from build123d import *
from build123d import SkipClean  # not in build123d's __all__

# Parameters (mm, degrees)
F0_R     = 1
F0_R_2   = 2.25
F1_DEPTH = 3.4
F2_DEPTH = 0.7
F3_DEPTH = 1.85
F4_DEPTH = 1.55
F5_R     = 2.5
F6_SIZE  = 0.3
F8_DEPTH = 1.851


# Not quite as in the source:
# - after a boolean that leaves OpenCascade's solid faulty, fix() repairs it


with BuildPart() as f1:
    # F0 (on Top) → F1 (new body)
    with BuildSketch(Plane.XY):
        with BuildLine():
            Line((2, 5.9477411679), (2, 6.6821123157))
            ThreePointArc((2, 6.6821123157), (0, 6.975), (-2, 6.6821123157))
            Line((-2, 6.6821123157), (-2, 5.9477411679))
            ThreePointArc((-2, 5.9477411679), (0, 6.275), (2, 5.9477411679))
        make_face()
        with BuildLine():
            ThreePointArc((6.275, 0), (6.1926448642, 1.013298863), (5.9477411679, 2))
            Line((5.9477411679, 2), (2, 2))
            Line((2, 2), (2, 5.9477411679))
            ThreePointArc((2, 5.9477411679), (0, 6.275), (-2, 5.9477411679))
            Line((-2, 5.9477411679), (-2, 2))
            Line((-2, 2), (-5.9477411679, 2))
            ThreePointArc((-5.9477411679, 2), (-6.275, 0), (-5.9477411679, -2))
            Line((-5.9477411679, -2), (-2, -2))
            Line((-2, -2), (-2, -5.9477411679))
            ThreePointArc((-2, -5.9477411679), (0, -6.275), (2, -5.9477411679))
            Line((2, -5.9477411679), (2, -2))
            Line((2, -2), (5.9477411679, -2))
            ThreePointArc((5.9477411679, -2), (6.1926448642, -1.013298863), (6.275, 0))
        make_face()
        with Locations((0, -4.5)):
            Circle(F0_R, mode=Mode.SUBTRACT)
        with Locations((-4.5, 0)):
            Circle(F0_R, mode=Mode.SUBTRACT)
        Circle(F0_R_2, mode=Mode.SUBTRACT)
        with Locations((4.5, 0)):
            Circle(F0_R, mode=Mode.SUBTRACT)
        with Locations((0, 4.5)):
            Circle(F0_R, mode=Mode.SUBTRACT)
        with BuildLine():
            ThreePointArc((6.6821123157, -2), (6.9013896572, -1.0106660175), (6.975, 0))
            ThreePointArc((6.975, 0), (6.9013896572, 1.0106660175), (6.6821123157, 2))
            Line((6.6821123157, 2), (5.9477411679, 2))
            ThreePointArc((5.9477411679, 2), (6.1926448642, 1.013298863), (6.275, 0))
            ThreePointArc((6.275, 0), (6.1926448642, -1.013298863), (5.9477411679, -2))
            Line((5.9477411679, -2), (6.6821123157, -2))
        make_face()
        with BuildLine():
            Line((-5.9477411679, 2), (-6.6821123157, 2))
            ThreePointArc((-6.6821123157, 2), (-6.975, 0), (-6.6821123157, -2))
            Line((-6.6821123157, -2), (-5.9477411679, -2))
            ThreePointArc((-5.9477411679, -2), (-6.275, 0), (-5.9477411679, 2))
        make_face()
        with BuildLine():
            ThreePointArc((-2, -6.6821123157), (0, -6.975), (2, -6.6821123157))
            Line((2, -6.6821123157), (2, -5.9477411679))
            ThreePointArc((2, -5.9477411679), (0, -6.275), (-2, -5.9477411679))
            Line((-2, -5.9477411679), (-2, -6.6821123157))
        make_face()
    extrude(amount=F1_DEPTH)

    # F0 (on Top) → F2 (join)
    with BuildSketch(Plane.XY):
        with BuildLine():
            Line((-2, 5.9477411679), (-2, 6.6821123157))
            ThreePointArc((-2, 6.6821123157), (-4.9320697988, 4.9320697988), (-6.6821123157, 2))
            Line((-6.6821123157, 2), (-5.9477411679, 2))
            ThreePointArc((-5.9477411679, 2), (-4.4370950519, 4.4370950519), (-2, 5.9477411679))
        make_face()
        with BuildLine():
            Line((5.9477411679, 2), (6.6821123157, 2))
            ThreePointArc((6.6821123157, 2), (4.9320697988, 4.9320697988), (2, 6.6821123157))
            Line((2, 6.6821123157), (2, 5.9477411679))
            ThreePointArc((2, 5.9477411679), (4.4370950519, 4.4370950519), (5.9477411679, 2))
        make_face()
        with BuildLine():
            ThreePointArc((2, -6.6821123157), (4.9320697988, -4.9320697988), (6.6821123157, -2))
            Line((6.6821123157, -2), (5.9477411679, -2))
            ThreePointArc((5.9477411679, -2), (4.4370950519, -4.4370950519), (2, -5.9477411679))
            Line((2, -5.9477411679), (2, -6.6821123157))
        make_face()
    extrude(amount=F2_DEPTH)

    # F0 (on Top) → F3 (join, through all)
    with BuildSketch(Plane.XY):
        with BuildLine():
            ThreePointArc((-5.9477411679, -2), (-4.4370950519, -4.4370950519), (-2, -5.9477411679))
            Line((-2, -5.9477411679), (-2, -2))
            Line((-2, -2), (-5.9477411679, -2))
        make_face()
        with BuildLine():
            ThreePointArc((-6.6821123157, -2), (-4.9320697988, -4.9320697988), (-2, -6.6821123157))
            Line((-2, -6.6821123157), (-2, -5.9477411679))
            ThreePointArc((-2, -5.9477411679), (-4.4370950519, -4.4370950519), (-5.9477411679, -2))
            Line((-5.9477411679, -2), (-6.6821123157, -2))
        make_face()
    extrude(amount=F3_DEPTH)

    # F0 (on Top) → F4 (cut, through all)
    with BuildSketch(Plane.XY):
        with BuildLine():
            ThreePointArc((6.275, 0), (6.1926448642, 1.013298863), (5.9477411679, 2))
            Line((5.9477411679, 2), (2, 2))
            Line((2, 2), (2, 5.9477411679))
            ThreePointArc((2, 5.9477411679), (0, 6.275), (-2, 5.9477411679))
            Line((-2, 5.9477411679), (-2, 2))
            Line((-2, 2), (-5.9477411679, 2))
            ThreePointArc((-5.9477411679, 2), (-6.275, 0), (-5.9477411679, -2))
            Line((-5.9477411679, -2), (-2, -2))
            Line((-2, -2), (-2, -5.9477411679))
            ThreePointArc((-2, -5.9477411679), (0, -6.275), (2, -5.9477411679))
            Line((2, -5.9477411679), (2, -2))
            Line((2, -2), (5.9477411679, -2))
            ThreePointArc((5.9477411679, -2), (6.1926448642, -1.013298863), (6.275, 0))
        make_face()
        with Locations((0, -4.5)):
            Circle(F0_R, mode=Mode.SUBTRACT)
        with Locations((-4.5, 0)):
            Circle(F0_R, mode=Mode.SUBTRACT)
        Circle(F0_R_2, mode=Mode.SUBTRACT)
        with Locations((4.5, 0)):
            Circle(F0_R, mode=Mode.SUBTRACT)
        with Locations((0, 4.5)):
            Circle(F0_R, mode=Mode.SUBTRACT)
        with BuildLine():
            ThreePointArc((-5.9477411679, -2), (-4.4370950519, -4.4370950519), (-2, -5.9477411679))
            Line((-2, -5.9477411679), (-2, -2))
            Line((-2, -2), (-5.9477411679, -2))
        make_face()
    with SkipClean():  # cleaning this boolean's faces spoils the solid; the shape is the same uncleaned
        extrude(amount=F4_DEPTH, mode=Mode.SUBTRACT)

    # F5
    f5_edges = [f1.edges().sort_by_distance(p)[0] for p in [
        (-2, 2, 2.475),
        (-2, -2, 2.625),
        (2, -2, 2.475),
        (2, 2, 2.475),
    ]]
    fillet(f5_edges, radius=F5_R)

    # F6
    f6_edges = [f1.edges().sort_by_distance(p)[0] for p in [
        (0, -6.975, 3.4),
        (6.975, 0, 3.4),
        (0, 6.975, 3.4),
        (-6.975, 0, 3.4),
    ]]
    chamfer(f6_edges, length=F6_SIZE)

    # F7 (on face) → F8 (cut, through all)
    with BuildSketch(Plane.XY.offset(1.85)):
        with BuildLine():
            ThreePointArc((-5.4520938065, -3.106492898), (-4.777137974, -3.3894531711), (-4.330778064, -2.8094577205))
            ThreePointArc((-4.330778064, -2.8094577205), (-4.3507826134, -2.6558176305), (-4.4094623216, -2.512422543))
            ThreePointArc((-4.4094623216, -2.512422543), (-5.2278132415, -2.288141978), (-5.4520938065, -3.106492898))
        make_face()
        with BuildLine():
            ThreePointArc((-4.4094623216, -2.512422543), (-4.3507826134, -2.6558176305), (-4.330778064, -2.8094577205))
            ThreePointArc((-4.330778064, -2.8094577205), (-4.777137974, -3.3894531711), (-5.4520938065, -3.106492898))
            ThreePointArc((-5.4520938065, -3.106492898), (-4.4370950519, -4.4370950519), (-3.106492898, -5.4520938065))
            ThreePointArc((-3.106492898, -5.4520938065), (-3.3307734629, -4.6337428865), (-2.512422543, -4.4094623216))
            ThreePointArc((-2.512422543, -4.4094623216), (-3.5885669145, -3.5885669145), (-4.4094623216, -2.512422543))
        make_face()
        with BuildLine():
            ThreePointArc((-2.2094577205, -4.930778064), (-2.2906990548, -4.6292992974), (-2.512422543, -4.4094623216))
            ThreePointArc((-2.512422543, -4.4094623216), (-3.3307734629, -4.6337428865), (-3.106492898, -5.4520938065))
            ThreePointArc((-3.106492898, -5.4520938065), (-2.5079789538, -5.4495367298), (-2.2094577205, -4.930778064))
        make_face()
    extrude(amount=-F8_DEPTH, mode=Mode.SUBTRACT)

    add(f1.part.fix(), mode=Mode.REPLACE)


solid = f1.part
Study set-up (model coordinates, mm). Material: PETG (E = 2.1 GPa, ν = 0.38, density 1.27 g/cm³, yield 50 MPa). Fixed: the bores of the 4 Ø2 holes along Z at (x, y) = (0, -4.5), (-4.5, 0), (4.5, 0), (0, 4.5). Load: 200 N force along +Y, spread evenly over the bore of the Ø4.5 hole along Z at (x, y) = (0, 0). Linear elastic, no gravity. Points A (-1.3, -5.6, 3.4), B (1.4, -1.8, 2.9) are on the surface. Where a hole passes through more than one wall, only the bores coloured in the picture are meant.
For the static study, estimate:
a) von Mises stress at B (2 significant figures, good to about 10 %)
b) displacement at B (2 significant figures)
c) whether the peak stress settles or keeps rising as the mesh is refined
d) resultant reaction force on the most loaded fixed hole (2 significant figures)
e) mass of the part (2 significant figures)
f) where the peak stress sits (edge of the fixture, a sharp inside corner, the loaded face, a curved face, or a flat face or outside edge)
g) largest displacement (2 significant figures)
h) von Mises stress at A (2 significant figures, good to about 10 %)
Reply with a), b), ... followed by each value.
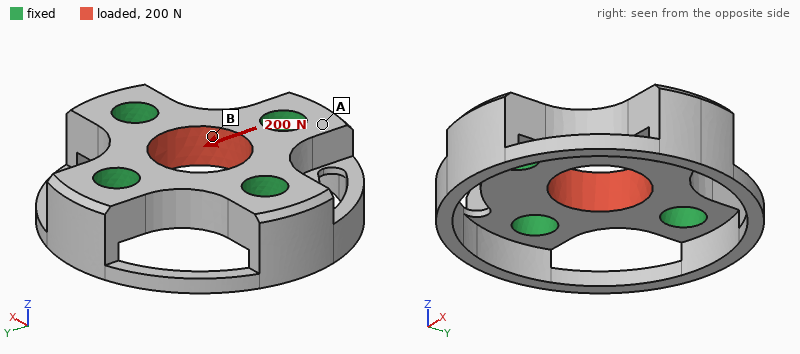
a) 11 MPa
b) 14 µm
c) keeps rising
d) 67 N
e) 0.21 g
f) edge of the fixture
g) 16 µm
h) 2.3 MPa
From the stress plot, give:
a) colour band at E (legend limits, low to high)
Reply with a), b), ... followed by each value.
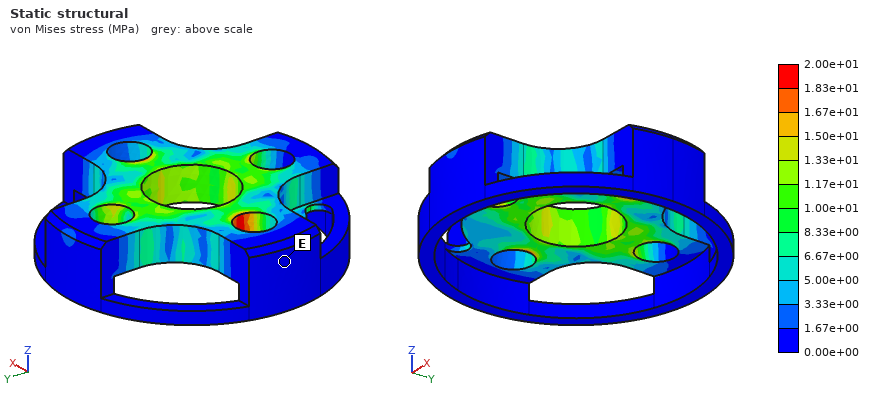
a) 0.00e+00 to 1.67e+00 MPa
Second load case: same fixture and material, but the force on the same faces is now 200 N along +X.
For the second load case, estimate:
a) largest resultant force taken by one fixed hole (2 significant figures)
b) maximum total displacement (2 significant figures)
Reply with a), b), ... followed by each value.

a) 67 N
b) 16 µm
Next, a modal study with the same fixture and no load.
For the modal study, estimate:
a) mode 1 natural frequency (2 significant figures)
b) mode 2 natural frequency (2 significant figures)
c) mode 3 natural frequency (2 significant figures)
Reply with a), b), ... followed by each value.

a) 15 kHz
b) 15 kHz
c) 16 kHz
